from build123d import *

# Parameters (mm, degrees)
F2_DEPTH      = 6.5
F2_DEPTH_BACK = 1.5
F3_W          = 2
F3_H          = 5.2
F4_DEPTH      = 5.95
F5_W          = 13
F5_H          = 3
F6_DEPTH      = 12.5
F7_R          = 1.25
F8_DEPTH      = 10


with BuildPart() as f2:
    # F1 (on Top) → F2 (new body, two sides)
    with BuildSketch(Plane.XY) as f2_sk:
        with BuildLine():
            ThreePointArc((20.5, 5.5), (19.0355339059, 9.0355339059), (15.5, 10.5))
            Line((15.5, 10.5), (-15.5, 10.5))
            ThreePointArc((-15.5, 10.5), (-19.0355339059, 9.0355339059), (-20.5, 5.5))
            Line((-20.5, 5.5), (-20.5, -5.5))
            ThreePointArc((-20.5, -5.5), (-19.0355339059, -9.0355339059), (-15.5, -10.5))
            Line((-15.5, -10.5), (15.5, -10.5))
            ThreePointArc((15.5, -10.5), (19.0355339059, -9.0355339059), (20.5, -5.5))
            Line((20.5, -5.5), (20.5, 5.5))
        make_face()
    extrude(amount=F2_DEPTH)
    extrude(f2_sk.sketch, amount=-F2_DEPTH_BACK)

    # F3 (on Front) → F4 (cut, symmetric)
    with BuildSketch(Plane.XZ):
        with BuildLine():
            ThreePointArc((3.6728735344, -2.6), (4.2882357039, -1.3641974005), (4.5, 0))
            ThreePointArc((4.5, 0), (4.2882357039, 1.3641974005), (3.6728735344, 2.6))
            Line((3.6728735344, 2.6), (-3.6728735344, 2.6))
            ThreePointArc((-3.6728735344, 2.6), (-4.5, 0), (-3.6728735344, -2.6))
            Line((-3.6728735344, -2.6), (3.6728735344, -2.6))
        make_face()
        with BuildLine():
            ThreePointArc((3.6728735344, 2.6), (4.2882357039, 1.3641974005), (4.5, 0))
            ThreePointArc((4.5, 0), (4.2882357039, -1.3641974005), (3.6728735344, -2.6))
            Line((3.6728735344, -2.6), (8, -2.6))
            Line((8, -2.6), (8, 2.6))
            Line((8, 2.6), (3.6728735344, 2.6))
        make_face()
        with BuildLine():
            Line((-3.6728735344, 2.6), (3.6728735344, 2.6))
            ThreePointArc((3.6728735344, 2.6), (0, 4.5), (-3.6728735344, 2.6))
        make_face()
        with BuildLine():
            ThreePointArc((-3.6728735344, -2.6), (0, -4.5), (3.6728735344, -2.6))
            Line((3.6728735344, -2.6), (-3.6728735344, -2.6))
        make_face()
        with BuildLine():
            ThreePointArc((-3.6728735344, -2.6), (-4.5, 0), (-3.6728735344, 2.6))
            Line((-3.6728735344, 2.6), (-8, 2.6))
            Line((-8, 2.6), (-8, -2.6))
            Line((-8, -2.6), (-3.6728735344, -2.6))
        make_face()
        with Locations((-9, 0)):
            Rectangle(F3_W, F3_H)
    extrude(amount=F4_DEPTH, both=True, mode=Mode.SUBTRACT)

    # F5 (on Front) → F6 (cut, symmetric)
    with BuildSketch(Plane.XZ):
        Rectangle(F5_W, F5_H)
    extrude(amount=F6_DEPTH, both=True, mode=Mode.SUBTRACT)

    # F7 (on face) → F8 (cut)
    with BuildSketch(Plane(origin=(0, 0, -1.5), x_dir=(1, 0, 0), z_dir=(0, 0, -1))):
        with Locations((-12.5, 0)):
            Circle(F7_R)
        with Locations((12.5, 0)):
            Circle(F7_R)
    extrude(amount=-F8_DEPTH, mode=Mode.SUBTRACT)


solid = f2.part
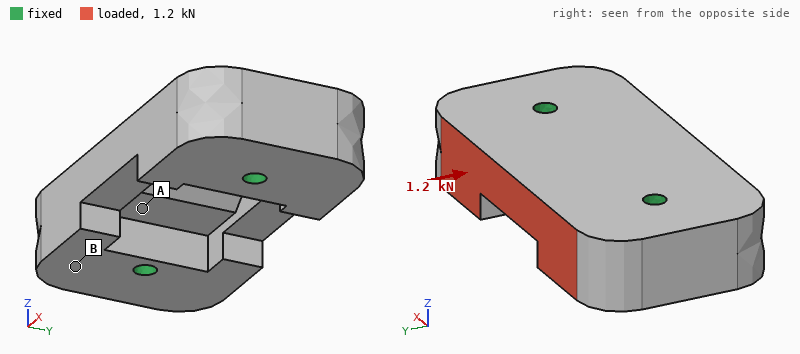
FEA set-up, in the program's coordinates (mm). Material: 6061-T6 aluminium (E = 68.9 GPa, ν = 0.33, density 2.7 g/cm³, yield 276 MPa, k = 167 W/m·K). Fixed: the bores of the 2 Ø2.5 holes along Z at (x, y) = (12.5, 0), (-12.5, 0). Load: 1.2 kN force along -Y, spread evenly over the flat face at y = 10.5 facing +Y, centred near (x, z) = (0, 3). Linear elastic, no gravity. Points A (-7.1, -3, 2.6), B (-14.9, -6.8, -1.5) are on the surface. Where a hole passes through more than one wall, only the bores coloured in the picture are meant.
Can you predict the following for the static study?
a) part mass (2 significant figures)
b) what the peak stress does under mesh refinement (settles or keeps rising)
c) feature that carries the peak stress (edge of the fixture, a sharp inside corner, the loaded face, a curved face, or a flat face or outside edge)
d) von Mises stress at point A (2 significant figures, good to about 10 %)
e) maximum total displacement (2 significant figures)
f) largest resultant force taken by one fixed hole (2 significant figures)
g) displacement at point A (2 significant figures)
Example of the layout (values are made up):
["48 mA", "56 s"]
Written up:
["14 g", "keeps rising", "edge of the fixture", "5.4 MPa", "3.1 µm", "610 N", "0.88 µm"]
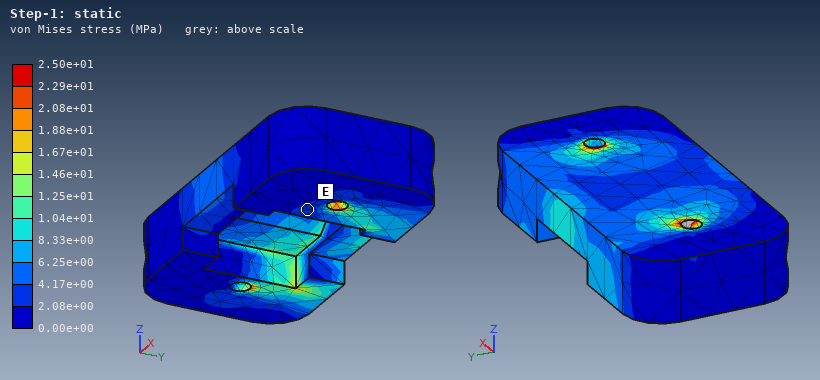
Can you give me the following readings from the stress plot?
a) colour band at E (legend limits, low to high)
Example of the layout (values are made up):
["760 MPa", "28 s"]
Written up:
["2.08e+00 to 4.17e+00 MPa"]
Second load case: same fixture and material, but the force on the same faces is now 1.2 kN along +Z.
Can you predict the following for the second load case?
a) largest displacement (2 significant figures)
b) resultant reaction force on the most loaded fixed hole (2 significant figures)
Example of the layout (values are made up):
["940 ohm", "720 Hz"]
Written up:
["22 µm", "640 N"]
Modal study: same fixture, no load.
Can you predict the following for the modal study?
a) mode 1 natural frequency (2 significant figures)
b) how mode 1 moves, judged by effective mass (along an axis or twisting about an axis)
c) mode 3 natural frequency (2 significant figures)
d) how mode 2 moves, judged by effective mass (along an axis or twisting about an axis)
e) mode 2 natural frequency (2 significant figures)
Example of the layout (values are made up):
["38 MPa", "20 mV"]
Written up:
["27 kHz", "twisting about X", "33 kHz", "along Z", "30 kHz"]
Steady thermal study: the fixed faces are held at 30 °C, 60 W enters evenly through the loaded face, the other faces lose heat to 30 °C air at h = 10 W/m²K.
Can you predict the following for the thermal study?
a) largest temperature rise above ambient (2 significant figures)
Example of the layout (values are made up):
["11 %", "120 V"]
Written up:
["26 K"]
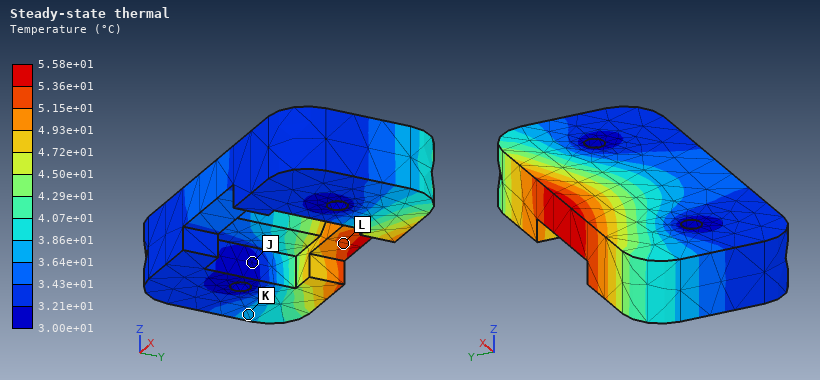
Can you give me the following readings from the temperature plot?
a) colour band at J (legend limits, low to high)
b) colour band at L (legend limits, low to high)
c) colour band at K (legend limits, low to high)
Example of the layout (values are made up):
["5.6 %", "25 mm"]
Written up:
["3.00e+01 to 3.21e+01 °C", "5.15e+01 to 5.36e+01 °C", "3.64e+01 to 3.86e+01 °C"]
